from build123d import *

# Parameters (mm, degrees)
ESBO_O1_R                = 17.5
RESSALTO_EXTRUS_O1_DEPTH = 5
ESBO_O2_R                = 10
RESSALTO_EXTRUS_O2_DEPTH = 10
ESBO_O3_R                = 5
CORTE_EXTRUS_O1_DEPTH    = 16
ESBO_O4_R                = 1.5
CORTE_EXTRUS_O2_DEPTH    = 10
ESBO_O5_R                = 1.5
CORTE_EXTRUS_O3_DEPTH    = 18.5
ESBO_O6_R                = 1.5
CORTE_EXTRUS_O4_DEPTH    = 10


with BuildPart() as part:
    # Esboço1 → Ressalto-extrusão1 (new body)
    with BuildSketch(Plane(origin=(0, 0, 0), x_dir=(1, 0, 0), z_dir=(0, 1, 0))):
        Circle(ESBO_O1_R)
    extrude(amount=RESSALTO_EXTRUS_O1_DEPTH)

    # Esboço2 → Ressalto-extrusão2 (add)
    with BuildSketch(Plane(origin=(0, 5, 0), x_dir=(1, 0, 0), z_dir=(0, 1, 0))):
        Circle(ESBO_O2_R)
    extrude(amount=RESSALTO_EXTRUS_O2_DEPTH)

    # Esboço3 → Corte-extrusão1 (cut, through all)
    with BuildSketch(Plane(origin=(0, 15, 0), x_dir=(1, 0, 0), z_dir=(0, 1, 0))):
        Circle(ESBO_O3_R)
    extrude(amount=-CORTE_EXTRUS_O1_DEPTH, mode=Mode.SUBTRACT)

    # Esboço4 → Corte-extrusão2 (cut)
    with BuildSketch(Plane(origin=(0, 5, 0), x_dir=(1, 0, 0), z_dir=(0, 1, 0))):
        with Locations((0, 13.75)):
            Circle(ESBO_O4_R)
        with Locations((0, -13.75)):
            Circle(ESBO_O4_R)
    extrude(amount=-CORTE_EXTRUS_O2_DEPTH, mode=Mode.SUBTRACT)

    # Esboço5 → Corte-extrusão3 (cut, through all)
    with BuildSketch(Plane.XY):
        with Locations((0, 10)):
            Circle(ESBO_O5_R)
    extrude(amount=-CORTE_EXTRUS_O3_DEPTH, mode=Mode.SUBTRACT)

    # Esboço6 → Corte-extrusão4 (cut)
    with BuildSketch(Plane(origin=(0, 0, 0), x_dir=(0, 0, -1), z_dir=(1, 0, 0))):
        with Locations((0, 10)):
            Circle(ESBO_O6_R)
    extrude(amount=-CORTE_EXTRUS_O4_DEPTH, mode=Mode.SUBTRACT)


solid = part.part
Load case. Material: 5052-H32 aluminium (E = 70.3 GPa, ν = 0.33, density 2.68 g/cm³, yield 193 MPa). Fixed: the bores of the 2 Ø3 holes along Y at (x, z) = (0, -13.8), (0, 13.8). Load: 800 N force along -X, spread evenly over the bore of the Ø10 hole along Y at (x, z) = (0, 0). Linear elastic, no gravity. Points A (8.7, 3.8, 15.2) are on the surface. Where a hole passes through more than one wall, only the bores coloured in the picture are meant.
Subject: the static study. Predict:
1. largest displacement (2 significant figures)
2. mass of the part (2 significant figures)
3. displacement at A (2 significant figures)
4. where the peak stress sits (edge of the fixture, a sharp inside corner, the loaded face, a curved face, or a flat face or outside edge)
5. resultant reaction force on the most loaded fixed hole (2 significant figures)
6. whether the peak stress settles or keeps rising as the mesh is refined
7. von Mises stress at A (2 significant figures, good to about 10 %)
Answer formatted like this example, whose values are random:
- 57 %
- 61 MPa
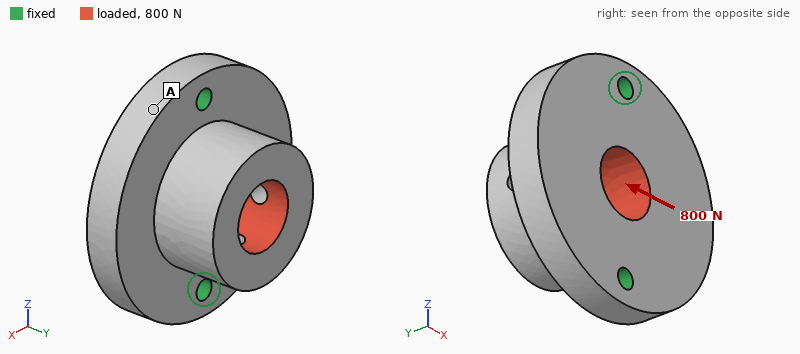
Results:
- 14 µm
- 18 g
- 4.0 µm
- edge of the fixture
- 400 N
- keeps rising
- 7.6 MPa
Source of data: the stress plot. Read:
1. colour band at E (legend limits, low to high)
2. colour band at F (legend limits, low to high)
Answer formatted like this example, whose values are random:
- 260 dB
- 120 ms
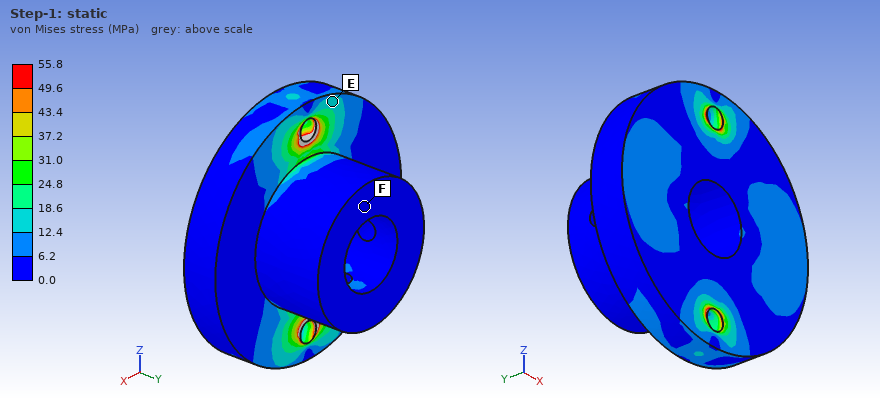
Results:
- 12.4 to 18.6 MPa
- 0.0 to 6.2 MPa
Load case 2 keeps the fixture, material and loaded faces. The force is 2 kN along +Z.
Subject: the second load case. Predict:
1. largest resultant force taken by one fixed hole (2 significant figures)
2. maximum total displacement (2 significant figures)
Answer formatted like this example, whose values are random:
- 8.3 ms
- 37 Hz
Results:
- 1.1 kN
- 7.0 µm
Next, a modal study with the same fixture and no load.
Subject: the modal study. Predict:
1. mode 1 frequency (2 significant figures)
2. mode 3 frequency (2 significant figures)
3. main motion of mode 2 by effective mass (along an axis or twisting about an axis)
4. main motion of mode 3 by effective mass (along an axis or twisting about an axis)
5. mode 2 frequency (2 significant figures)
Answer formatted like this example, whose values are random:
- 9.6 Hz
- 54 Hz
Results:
- 9200 Hz
- 29 kHz
- along Y
- along Z
- 18 kHz
